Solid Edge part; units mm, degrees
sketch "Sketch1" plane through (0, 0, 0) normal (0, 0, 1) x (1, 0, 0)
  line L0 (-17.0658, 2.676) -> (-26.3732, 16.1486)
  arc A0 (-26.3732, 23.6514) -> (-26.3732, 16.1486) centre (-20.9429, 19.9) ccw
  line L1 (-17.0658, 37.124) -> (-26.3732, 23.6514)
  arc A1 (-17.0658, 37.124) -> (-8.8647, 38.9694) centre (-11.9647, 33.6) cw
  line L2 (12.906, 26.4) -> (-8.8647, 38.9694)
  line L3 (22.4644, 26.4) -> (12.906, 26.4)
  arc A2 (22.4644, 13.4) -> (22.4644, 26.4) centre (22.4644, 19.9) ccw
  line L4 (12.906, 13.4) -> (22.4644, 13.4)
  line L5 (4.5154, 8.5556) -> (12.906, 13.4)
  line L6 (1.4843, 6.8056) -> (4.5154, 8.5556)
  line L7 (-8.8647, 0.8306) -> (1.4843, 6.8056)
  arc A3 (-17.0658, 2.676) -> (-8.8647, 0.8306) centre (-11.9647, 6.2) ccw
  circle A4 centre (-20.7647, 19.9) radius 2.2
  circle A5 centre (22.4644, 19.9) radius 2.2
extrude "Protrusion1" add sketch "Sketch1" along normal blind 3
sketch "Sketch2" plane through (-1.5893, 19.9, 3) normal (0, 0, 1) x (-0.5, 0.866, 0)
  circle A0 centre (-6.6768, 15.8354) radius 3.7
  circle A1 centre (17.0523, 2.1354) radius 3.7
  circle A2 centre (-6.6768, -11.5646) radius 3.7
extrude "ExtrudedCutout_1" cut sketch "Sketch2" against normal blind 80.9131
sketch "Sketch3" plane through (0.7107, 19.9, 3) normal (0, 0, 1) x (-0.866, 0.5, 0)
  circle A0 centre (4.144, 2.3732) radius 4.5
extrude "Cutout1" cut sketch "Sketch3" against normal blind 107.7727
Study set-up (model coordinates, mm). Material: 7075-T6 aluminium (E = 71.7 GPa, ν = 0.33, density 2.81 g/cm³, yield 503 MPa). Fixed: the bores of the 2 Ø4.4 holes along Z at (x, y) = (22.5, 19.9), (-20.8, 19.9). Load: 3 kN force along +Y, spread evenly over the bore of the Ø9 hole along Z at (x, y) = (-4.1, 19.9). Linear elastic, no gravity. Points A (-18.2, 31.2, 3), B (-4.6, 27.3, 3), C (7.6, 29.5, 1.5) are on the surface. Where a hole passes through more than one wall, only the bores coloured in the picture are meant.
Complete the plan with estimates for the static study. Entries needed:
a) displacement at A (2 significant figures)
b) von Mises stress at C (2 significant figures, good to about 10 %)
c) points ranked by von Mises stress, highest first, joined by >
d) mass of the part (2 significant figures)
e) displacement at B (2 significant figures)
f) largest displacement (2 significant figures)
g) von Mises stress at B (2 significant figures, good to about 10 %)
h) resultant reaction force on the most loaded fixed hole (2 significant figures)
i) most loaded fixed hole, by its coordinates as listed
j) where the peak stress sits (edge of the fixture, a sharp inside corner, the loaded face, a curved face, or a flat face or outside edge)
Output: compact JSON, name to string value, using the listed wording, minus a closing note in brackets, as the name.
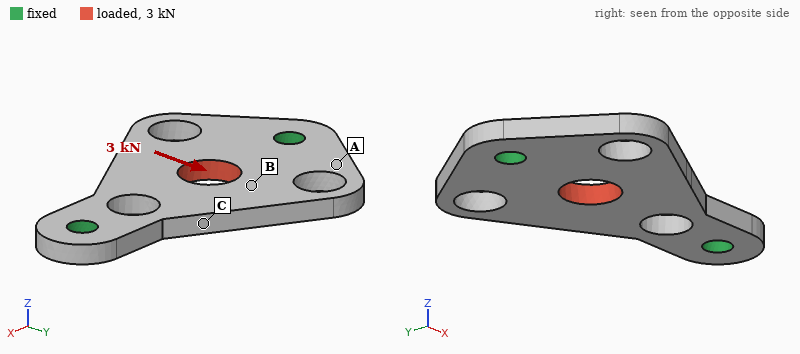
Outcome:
{"displacement at A": "17 µm", "von Mises stress at C": "120 MPa", "points ranked by von Mises stress, highest first, joined by >": "C > B > A", "mass of the part": "8.8 g", "displacement at B": "36 µm", "largest displacement": "44 µm", "von Mises stress at B": "56 MPa", "resultant reaction force on the most loaded fixed hole": "1.9 kN", "most loaded fixed hole, by its coordinates as listed": "(-20.8, 19.9)", "where the peak stress sits": "edge of the fixture"}
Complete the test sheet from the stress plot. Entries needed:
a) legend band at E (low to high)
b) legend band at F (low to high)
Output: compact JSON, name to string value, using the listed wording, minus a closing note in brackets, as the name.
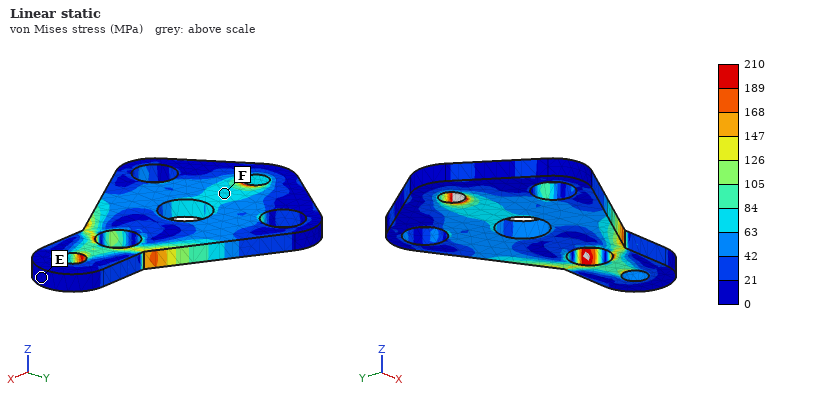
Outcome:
{"legend band at E": "0 to 21 MPa", "legend band at F": "63 to 84 MPa"}
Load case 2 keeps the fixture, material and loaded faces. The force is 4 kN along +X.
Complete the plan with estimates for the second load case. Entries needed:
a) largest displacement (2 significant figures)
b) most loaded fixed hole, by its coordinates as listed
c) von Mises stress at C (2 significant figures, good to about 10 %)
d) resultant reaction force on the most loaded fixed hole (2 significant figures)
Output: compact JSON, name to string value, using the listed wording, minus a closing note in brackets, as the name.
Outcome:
{"largest displacement": "19 µm", "most loaded fixed hole, by its coordinates as listed": "(-20.8, 19.9)", "von Mises stress at C": "13 MPa", "resultant reaction force on the most loaded fixed hole": "2.7 kN"}
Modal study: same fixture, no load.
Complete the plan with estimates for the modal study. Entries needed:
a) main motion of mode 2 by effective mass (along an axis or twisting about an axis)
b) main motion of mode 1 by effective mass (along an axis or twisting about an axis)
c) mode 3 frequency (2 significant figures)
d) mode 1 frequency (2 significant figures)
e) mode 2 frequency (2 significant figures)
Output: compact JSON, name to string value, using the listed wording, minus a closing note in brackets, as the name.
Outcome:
{"main motion of mode 2 by effective mass": "along Z", "main motion of mode 1 by effective mass": "twisting about X", "mode 3 frequency": "12 kHz", "mode 1 frequency": "6000 Hz", "mode 2 frequency": "6700 Hz"}
